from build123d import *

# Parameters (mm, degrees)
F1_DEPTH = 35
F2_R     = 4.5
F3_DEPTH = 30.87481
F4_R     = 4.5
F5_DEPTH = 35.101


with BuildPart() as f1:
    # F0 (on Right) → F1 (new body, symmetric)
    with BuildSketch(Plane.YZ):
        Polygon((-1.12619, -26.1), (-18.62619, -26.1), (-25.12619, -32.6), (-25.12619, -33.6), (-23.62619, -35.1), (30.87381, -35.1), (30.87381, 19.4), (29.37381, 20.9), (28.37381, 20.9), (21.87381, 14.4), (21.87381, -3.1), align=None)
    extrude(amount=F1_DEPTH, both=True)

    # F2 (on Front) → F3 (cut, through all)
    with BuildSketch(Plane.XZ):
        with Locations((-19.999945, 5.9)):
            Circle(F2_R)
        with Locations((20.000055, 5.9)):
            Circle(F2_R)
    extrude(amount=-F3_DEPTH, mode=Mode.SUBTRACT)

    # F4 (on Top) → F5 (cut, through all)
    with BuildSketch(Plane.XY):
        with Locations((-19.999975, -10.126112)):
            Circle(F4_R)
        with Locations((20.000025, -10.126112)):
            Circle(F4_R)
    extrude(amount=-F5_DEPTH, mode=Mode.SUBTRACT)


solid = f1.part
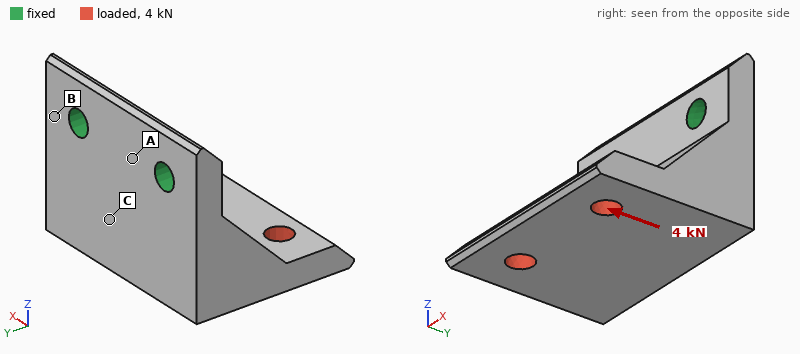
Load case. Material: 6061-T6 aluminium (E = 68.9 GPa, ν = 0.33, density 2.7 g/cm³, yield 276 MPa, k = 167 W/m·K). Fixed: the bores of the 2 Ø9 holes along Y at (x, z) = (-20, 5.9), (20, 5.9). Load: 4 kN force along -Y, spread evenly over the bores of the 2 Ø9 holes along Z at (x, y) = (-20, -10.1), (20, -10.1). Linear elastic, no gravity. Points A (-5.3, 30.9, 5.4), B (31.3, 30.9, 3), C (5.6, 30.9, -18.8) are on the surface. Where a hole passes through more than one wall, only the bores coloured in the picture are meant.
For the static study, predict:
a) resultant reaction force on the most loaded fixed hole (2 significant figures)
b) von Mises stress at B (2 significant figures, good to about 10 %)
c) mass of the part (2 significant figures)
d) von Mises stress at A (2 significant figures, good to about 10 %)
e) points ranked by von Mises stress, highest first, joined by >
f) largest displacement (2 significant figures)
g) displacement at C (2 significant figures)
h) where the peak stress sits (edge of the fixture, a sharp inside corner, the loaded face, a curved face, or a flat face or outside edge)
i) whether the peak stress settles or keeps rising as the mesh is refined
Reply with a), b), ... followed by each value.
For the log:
a) 2.0 kN
b) 74 MPa
c) 210 g
d) 46 MPa
e) B > A > C
f) 0.33 mm
g) 0.100 mm
h) edge of the fixture
i) keeps rising
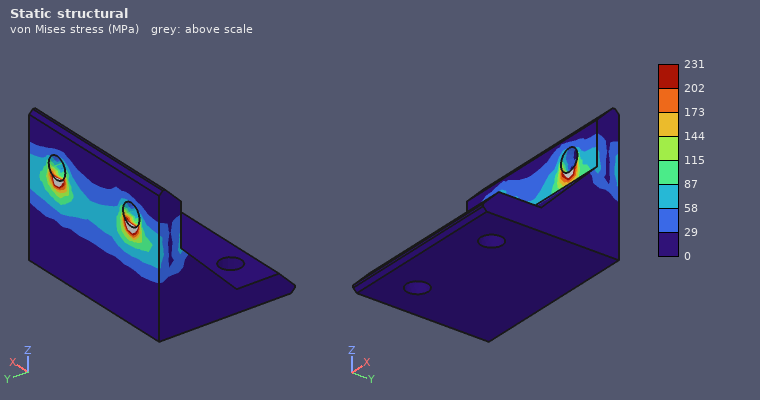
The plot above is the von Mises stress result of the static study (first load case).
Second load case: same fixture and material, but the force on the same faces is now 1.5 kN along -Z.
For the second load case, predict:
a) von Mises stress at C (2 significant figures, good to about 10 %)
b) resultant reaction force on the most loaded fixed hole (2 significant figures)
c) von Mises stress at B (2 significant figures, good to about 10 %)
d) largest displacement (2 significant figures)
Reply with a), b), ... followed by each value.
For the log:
a) 9.0 MPa
b) 770 N
c) 31 MPa
d) 0.17 mm
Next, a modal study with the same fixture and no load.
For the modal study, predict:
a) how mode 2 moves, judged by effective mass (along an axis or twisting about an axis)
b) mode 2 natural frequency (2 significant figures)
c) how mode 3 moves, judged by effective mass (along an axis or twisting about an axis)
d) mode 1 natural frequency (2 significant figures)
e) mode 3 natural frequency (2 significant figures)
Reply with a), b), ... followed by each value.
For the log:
a) along X
b) 4500 Hz
c) along X
d) 1800 Hz
e) 7400 Hz
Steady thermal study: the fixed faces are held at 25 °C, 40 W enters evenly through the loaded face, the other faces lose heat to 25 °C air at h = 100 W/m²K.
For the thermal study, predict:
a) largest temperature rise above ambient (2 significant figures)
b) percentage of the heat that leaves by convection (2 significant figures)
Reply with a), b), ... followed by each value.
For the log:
a) 16 K
b) 26 %
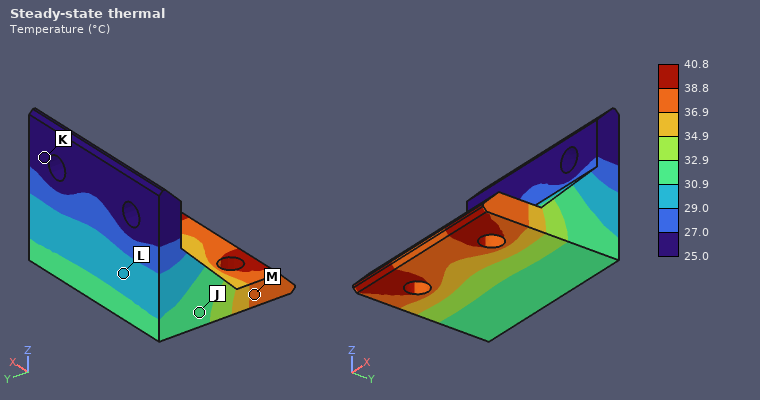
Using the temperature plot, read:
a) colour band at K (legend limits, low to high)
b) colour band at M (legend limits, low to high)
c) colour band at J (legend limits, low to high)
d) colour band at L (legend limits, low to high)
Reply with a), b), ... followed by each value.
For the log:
a) 25.0 to 27.0 °C
b) 36.9 to 38.8 °C
c) 30.9 to 32.9 °C
d) 29.0 to 30.9 °C
